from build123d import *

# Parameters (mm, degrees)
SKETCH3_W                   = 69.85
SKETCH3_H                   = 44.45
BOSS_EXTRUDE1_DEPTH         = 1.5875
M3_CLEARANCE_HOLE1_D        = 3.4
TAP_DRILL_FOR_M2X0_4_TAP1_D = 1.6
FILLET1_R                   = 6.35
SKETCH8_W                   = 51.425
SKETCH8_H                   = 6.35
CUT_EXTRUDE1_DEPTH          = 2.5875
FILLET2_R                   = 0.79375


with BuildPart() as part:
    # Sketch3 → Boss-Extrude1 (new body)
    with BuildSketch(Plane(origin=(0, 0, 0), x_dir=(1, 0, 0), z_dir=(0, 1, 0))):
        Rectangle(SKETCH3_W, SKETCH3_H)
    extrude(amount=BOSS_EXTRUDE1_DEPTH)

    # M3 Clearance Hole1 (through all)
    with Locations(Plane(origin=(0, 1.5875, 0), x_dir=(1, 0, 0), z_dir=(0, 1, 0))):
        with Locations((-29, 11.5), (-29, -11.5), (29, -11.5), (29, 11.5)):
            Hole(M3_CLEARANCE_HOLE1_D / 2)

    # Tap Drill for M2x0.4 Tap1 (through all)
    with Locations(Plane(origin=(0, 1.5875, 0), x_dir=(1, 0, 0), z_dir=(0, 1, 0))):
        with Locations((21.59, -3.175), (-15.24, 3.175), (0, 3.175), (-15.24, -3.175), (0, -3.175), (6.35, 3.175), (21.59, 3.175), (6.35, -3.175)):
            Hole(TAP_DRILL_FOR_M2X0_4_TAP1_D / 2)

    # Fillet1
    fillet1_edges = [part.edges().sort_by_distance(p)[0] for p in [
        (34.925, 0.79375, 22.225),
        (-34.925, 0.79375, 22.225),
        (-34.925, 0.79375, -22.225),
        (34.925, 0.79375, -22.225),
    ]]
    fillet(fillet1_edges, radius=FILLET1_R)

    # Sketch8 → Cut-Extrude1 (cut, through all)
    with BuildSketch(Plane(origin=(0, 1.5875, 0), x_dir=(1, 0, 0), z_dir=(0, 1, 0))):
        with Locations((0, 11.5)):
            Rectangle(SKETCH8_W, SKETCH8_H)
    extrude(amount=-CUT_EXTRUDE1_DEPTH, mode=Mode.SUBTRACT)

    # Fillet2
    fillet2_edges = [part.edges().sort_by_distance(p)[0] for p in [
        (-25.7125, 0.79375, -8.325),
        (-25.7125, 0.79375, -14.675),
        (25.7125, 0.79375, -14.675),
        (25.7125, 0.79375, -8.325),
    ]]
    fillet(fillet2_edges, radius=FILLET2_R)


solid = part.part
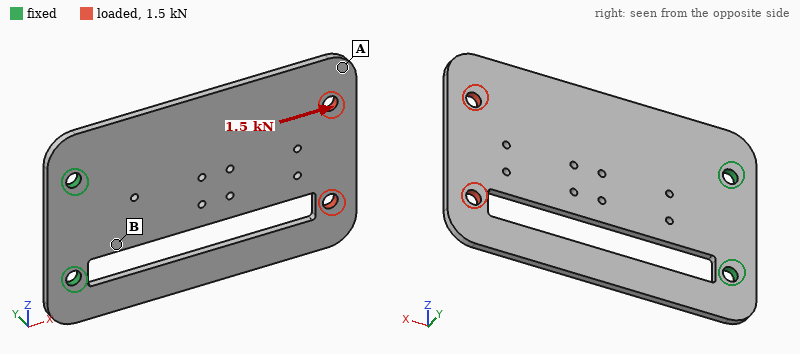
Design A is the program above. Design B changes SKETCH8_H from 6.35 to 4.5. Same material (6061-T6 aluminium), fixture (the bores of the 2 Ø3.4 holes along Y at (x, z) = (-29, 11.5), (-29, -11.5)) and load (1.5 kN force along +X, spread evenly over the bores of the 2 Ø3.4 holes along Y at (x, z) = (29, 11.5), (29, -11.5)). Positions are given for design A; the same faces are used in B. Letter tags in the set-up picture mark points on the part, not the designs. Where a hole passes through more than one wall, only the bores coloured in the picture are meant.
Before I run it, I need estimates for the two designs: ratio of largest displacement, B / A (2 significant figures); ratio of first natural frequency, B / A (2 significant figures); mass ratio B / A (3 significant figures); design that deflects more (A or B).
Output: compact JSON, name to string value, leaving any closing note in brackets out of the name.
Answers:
{"ratio of largest displacement, B / A": "0.83", "ratio of first natural frequency, B / A": "1.0", "mass ratio B / A": "1.04", "design that deflects more": "A"}
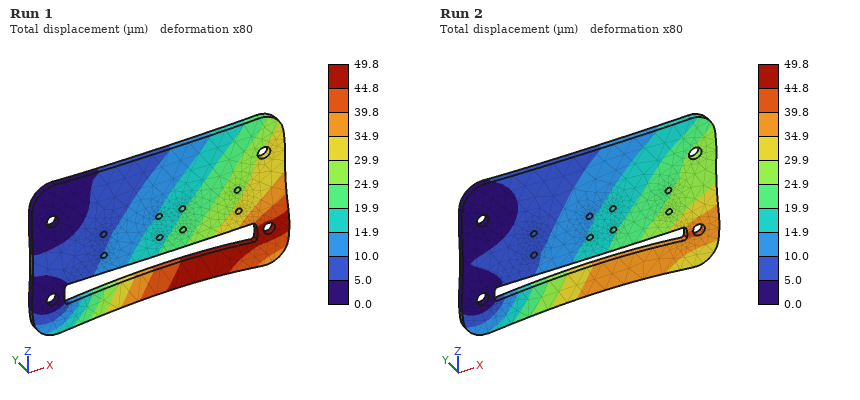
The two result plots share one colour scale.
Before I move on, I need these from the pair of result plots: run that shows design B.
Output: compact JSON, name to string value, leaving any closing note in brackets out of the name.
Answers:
{"run that shows design B": "Run 2"}
